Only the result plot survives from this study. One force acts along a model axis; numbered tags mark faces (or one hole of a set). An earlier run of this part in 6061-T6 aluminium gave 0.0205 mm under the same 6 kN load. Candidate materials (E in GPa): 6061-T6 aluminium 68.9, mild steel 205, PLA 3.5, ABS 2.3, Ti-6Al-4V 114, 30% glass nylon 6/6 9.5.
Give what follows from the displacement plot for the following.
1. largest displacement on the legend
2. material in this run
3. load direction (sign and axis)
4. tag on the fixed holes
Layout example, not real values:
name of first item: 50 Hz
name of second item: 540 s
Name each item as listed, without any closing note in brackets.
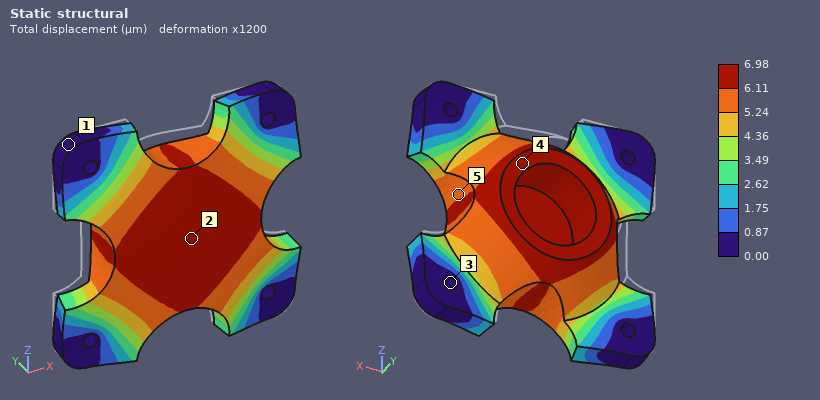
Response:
largest displacement on the legend: 6.98 µm
material in this run: mild steel
load direction: -Y
tag on the fixed holes: 3
